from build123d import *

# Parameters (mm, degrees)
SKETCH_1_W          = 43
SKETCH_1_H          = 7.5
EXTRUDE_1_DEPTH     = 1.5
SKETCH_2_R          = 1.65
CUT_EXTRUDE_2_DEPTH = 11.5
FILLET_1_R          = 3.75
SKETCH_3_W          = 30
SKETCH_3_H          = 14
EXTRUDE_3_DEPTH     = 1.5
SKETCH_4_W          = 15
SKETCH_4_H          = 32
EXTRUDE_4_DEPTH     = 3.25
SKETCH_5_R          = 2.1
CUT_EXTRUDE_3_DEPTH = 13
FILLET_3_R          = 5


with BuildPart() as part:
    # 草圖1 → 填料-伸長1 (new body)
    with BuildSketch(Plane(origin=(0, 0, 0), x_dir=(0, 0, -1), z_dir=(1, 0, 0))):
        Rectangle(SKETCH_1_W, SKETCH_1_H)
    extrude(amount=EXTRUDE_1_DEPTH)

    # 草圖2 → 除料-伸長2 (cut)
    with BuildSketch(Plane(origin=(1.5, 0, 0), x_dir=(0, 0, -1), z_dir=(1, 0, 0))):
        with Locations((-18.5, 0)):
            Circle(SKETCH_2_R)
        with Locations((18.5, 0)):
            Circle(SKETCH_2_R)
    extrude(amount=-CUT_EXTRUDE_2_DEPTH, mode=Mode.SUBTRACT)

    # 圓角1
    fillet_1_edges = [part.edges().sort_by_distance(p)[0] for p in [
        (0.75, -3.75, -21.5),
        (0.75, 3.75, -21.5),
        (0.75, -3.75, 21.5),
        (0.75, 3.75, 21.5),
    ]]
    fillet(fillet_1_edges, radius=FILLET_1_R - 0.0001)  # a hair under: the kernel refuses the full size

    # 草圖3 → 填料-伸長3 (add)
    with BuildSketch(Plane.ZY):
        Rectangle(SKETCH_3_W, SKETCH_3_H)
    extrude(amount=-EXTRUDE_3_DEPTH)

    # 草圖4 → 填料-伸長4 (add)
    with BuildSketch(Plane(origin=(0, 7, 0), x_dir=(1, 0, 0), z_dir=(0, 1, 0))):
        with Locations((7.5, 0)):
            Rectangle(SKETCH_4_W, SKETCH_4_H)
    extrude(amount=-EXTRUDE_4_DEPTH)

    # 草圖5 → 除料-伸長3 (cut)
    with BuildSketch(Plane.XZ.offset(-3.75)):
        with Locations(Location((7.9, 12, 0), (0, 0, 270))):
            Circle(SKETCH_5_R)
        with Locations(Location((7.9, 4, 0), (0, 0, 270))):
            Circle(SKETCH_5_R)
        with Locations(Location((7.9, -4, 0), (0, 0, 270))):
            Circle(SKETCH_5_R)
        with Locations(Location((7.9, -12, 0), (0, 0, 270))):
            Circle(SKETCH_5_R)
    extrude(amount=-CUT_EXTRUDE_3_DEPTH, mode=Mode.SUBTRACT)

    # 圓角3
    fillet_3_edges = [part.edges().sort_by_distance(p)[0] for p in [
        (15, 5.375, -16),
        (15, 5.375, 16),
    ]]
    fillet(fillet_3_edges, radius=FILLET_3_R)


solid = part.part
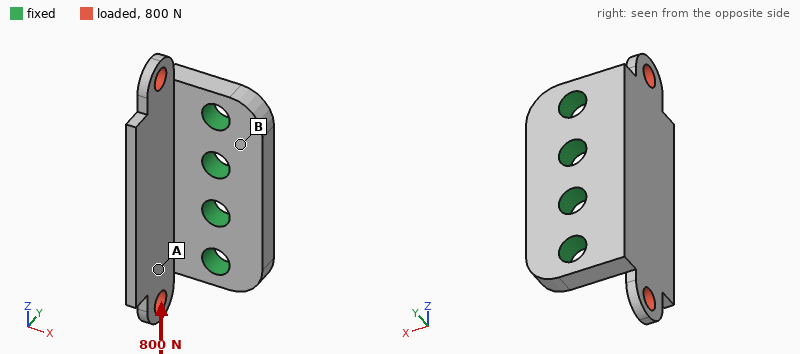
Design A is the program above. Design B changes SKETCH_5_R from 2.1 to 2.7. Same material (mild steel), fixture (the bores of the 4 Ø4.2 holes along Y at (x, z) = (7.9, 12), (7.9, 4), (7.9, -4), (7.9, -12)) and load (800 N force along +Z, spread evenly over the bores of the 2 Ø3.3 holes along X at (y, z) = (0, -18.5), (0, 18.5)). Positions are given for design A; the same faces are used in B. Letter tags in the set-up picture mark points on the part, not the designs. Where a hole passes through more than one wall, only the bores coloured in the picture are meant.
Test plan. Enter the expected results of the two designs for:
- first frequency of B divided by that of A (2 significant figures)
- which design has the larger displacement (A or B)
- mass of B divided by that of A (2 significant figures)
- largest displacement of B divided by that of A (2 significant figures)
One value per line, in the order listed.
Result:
1.0
A
0.94
0.88
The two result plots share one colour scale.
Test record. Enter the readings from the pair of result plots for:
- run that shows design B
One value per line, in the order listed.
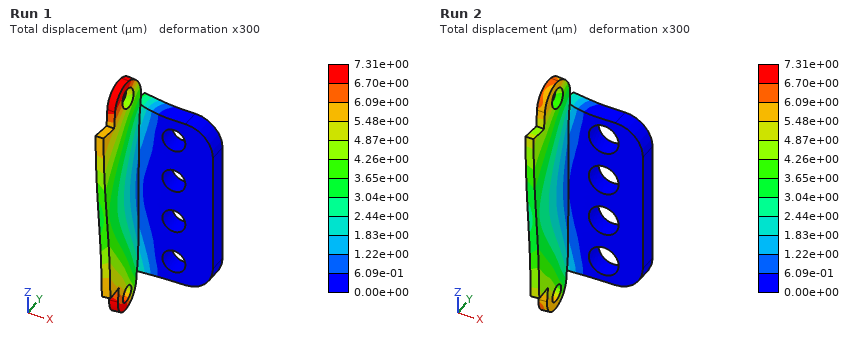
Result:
Run 2
